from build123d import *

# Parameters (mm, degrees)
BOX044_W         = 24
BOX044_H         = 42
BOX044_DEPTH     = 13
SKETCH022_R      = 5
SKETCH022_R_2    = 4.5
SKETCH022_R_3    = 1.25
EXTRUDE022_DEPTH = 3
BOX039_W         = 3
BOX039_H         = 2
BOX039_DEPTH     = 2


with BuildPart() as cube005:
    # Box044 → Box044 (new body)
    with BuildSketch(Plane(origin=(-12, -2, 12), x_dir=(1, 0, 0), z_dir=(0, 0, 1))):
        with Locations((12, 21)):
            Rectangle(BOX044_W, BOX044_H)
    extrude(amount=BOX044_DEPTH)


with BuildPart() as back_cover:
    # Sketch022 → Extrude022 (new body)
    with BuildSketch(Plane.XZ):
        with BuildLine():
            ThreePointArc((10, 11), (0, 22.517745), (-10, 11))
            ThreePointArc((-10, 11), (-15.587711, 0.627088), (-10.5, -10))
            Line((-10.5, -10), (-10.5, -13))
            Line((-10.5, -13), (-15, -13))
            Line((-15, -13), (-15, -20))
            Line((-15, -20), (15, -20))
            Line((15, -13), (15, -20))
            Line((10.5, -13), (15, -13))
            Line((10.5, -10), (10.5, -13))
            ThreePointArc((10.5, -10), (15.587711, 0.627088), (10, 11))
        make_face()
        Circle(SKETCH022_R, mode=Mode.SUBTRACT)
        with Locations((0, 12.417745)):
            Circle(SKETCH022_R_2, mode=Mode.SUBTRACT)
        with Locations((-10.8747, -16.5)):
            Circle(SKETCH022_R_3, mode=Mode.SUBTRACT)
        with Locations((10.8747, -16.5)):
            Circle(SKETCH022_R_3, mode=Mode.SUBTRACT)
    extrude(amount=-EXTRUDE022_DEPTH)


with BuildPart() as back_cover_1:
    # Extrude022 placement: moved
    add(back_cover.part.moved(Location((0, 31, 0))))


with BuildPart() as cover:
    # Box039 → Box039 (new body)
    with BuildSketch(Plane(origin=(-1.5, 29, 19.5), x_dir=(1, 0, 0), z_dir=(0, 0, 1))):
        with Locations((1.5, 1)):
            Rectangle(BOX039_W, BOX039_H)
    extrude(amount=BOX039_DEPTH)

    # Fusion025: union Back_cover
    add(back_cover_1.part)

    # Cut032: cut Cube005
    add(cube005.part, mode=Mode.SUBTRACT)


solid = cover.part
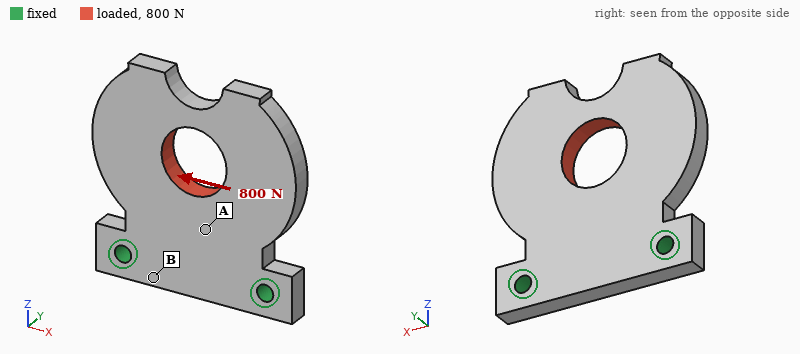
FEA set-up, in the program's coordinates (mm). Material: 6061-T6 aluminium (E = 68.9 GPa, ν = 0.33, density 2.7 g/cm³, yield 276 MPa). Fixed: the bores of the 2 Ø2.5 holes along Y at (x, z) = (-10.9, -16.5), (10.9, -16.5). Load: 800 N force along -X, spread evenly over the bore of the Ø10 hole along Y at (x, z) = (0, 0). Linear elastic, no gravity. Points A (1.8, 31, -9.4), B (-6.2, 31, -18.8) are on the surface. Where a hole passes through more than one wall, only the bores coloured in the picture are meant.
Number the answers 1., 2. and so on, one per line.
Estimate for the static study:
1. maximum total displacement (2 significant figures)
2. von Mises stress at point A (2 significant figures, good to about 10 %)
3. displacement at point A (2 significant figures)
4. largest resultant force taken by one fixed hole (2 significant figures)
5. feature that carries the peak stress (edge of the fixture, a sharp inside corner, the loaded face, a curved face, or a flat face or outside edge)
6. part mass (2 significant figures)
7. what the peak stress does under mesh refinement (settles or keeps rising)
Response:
1. 35 µm
2. 37 MPa
3. 5.4 µm
4. 740 N
5. a sharp inside corner
6. 6.2 g
7. keeps rising
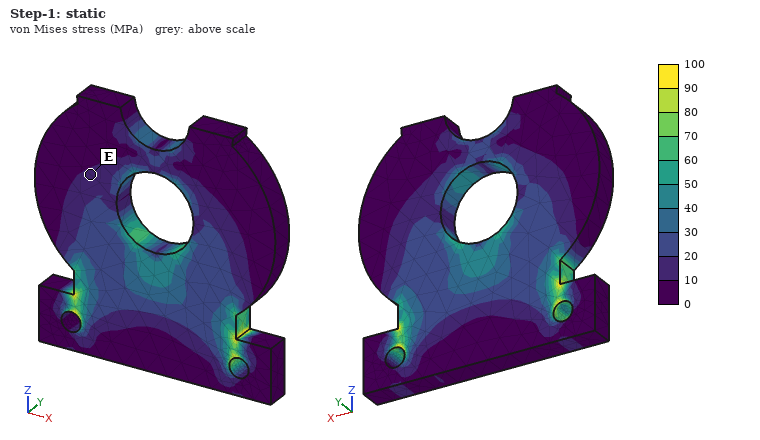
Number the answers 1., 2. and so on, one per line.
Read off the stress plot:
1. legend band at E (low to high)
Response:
1. 10 to 20 MPa
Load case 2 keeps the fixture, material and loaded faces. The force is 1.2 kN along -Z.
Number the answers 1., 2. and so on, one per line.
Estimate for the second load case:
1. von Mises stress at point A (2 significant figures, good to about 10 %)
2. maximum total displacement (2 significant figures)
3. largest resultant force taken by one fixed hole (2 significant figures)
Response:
1. 9.3 MPa
2. 14 µm
3. 630 N
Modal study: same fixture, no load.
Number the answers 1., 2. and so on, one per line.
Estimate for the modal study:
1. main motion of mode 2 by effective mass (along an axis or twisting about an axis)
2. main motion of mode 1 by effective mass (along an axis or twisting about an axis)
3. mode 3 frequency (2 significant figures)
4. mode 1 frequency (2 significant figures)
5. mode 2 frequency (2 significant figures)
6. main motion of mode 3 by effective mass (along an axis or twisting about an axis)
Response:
1. twisting about Z
2. along Y
3. 13 kHz
4. 2700 Hz
5. 5900 Hz
6. along X
